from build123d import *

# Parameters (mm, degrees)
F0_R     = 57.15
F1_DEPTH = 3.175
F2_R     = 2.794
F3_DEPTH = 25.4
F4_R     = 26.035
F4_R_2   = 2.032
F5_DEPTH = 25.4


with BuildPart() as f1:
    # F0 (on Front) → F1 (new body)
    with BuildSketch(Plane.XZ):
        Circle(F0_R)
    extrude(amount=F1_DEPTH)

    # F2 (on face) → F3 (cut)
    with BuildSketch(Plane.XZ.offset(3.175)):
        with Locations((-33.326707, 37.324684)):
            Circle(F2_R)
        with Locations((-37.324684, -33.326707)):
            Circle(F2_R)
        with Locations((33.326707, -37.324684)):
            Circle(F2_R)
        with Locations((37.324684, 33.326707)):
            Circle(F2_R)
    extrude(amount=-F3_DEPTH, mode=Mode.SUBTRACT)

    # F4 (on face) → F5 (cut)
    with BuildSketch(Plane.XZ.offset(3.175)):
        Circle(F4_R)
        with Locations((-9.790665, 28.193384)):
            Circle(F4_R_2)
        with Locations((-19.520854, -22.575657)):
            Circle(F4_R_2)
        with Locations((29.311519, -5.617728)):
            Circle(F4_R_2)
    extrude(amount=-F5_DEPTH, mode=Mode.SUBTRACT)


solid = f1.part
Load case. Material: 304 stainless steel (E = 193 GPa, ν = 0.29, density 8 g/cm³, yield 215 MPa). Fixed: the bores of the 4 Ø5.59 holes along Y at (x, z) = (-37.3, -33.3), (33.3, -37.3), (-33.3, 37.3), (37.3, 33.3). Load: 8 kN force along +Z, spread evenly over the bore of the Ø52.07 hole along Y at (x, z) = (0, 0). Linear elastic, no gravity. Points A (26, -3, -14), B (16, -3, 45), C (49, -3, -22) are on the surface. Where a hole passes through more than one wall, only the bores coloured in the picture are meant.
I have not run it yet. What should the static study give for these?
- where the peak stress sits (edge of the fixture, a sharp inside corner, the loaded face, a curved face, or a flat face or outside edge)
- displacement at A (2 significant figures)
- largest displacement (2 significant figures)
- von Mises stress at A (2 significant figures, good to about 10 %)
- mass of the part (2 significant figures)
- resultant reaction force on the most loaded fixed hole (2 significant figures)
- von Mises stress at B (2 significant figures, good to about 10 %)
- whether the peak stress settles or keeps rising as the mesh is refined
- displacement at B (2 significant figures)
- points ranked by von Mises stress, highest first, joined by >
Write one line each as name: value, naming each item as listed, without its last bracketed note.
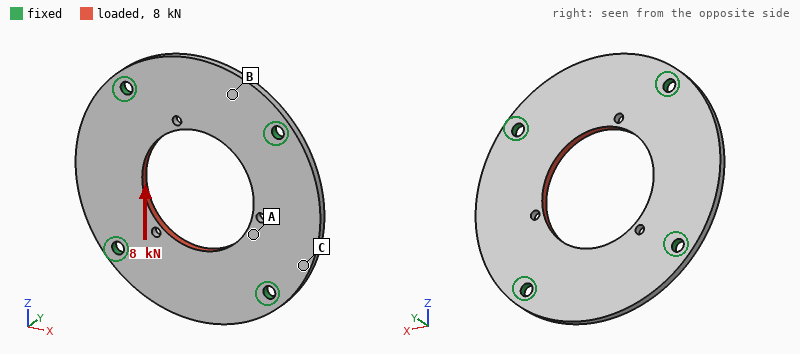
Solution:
where the peak stress sits: edge of the fixture
displacement at A: 3.5 µm
largest displacement: 7.3 µm
von Mises stress at A: 30 MPa
mass of the part: 200 g
resultant reaction force on the most loaded fixed hole: 2.0 kN
von Mises stress at B: 15 MPa
whether the peak stress settles or keeps rising as the mesh is refined: keeps rising
displacement at B: 5.2 µm
points ranked by von Mises stress, highest first, joined by >: A > B > C
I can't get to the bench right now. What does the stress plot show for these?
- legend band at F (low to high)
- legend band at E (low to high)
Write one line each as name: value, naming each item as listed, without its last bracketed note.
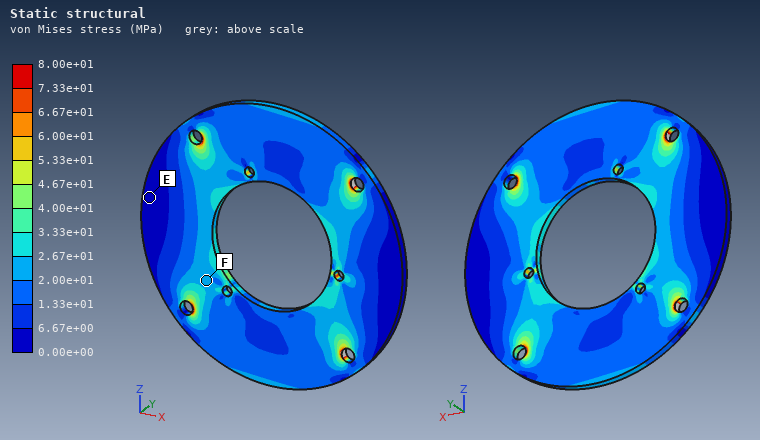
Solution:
legend band at F: 2.00e+01 to 2.67e+01 MPa
legend band at E: 0.00e+00 to 6.67e+00 MPa
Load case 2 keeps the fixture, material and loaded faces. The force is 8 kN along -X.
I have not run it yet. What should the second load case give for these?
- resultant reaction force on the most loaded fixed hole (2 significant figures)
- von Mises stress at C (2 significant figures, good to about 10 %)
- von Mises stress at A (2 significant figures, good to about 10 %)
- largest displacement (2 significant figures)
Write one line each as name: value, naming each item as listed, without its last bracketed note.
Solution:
resultant reaction force on the most loaded fixed hole: 2.0 kN
von Mises stress at C: 17 MPa
von Mises stress at A: 13 MPa
largest displacement: 7.7 µm
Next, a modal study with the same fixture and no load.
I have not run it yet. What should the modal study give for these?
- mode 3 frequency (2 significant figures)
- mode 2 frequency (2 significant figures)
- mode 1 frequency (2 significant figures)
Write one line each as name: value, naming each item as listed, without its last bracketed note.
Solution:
mode 3 frequency: 2800 Hz
mode 2 frequency: 2800 Hz
mode 1 frequency: 2600 Hz
